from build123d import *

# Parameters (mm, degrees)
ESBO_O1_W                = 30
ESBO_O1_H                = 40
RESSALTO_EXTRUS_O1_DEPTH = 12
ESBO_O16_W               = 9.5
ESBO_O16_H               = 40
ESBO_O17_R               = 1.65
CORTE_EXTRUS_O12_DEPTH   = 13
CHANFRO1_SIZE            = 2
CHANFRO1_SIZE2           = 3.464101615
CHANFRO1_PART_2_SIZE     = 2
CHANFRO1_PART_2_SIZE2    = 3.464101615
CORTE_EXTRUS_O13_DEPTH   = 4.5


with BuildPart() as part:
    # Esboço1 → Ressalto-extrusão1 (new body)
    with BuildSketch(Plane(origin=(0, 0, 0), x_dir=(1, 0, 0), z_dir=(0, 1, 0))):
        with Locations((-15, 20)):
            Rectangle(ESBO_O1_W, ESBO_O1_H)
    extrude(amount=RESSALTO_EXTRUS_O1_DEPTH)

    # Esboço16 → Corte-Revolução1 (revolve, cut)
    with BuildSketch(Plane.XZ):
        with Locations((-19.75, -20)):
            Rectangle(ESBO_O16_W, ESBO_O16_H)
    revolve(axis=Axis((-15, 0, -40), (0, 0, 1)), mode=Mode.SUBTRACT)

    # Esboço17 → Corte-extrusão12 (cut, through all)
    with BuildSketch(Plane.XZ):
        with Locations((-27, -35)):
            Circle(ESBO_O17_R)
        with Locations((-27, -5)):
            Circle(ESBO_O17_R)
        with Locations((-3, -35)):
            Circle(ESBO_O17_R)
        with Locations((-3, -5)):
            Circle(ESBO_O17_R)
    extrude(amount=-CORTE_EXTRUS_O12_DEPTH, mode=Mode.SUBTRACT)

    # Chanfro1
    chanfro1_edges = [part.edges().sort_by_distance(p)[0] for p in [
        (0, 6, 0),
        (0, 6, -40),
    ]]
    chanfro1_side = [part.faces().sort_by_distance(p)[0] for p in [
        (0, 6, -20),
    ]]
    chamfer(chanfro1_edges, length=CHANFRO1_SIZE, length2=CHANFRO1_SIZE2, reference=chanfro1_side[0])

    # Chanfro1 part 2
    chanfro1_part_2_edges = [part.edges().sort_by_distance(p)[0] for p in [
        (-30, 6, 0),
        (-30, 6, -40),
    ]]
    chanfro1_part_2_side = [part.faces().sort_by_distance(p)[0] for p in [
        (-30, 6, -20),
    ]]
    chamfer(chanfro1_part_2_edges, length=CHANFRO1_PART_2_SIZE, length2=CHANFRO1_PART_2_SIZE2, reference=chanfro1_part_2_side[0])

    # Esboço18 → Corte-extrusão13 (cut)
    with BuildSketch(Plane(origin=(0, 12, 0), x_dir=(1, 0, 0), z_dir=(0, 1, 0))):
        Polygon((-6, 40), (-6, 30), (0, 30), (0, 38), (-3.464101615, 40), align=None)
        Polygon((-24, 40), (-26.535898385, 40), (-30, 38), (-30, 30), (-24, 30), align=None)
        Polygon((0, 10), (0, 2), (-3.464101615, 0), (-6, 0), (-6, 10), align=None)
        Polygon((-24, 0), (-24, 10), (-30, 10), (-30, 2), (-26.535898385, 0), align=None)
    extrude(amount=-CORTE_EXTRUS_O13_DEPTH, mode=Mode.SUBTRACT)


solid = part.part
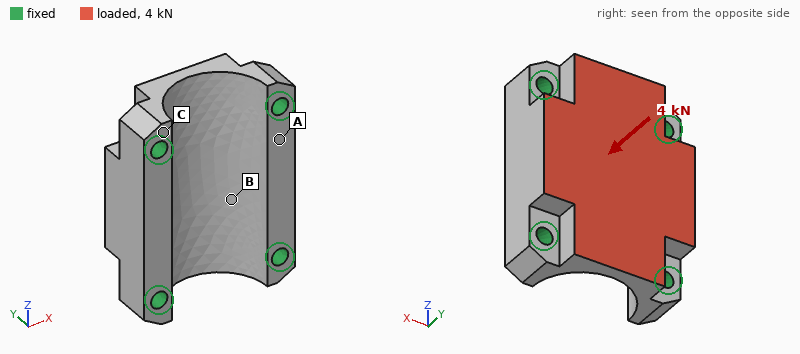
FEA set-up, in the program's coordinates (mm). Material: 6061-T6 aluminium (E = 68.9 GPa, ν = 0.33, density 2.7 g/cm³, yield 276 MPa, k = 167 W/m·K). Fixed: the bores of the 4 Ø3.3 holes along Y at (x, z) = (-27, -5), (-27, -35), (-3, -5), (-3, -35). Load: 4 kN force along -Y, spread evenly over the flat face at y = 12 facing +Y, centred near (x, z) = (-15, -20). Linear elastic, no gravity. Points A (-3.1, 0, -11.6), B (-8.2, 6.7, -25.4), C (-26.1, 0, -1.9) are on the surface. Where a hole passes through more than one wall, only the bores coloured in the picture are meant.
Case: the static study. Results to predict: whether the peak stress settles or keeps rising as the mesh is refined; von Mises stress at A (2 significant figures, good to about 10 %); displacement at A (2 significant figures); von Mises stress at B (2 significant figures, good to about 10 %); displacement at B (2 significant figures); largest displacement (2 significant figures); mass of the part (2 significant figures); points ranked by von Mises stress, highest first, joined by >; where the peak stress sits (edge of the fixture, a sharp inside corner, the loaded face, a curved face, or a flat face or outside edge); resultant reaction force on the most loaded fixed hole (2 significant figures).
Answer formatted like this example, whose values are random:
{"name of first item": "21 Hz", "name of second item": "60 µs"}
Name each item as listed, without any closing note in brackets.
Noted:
{"whether the peak stress settles or keeps rising as the mesh is refined": "keeps rising", "von Mises stress at A": "11 MPa", "displacement at A": "4.6 µm", "von Mises stress at B": "19 MPa", "displacement at B": "7.5 µm", "largest displacement": "12 µm", "mass of the part": "20 g", "points ranked by von Mises stress, highest first, joined by >": "B > A > C", "where the peak stress sits": "edge of the fixture", "resultant reaction force on the most loaded fixed hole": "1.2 kN"}
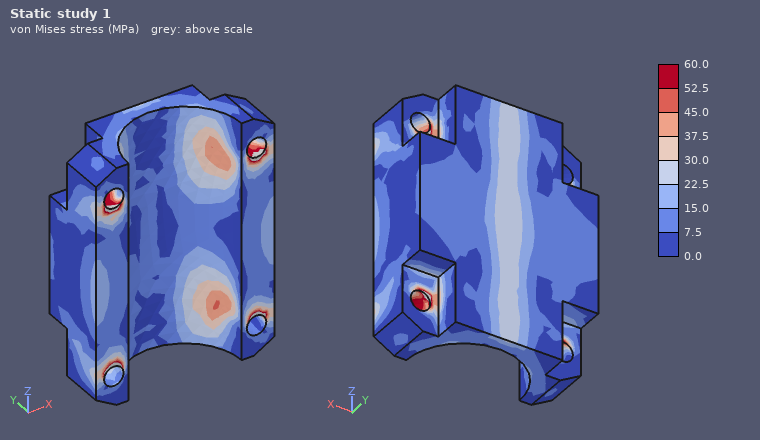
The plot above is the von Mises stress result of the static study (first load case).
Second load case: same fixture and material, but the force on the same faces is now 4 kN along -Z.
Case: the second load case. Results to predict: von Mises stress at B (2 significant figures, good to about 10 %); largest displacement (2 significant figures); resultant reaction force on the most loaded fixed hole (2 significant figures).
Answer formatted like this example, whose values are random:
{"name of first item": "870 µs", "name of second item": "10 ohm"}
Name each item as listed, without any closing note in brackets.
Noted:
{"von Mises stress at B": "21 MPa", "largest displacement": "9.0 µm", "resultant reaction force on the most loaded fixed hole": "1.1 kN"}
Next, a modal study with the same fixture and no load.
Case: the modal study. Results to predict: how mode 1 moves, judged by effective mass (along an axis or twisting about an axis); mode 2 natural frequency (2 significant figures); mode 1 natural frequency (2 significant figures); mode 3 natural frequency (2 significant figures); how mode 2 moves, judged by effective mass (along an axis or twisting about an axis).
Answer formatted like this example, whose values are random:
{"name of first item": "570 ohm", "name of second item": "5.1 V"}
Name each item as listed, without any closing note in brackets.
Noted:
{"how mode 1 moves, judged by effective mass": "along X", "mode 2 natural frequency": "31 kHz", "mode 1 natural frequency": "29 kHz", "mode 3 natural frequency": "35 kHz", "how mode 2 moves, judged by effective mass": "along Y"}
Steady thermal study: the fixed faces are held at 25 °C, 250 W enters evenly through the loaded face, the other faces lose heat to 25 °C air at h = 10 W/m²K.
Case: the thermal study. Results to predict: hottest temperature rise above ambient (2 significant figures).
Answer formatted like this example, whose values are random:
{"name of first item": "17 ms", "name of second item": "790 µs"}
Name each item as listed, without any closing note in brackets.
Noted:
{"hottest temperature rise above ambient": "59 K"}
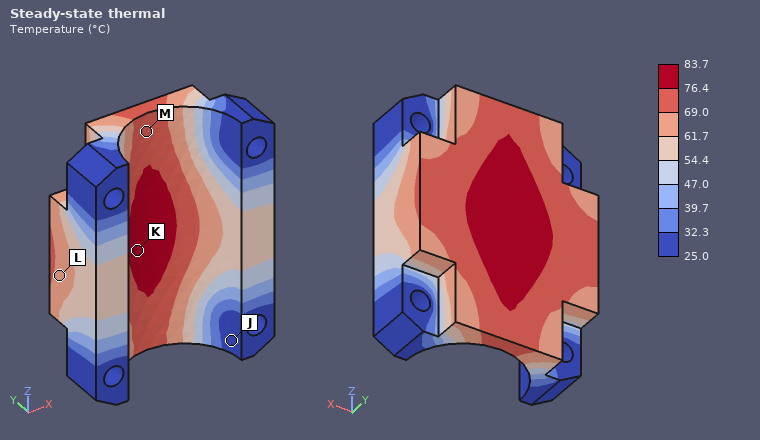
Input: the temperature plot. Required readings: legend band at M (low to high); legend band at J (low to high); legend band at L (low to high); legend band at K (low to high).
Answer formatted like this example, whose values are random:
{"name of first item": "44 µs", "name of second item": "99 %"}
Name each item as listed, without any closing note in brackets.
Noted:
{"legend band at M": "69.0 to 76.4 °C", "legend band at J": "25.0 to 32.3 °C", "legend band at L": "61.7 to 69.0 °C", "legend band at K": "76.4 to 83.7 °C"}
